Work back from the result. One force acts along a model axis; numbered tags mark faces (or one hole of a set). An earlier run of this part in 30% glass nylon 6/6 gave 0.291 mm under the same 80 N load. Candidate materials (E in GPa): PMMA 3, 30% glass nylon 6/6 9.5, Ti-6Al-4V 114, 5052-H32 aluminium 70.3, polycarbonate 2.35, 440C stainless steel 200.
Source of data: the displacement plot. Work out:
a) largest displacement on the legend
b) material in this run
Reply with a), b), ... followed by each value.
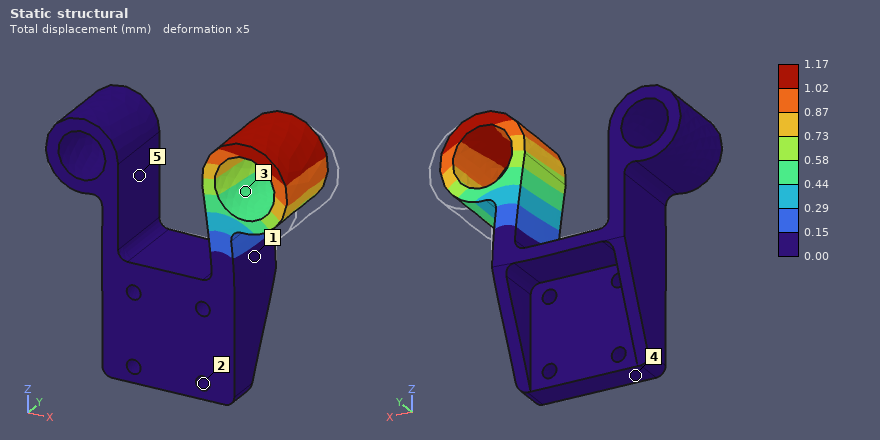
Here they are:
a) 1.17 mm
b) polycarbonate
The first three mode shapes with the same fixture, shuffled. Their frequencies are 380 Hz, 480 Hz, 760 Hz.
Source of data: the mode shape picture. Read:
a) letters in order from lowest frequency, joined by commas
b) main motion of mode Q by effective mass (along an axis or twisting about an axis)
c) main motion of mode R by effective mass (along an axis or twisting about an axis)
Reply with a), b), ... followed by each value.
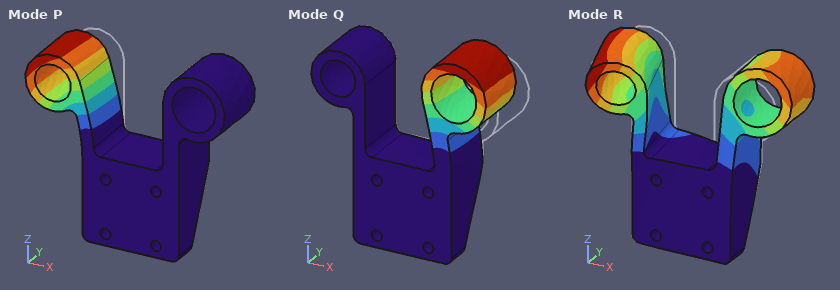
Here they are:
a) P, Q, R
b) along X
c) twisting about Z
